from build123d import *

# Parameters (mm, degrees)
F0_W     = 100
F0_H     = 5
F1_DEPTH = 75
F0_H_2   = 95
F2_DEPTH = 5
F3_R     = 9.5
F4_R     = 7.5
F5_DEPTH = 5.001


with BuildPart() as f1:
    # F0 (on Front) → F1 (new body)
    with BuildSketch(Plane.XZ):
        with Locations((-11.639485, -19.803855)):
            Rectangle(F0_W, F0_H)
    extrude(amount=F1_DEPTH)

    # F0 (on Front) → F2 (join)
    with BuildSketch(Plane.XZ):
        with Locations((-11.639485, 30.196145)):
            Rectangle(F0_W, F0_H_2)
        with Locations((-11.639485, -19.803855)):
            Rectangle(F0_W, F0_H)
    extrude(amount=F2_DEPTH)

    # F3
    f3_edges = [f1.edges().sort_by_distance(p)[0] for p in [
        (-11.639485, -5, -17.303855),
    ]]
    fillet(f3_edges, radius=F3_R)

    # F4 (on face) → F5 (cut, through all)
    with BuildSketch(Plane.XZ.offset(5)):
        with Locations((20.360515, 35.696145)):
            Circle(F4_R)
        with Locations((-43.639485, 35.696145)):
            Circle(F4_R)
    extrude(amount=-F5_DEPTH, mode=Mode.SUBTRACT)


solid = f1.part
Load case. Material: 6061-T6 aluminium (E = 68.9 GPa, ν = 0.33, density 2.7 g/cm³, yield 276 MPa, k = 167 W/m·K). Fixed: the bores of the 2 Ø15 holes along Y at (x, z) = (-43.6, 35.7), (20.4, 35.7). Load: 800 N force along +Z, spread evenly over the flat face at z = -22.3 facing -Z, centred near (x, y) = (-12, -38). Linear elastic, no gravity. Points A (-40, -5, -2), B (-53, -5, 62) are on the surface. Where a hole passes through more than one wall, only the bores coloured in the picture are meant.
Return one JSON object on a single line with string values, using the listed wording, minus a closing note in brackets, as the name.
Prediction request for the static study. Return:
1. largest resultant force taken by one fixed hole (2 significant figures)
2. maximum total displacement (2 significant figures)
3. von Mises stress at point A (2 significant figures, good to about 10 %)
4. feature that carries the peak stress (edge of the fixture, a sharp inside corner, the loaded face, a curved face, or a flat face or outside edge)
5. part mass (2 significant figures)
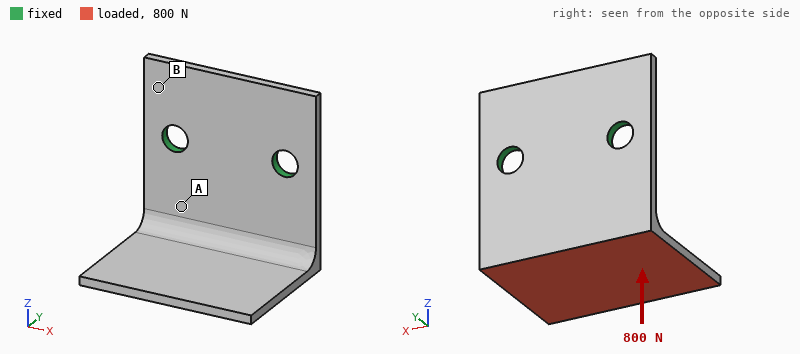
{"largest resultant force taken by one fixed hole": "410 N", "maximum total displacement": "1.6 mm", "von Mises stress at point A": "61 MPa", "feature that carries the peak stress": "a flat face or outside edge", "part mass": "230 g"}
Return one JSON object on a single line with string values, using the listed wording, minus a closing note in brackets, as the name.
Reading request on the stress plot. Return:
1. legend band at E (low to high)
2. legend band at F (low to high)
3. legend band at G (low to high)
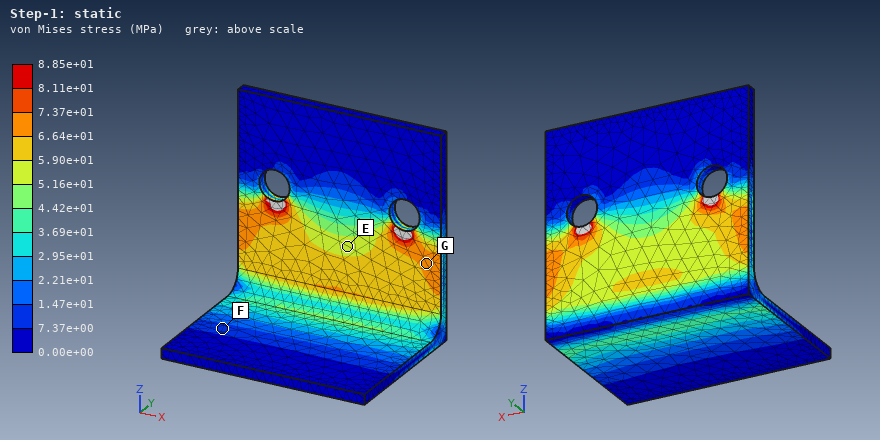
{"legend band at E": "5.16e+01 to 5.90e+01 MPa", "legend band at F": "7.37e+00 to 1.47e+01 MPa", "legend band at G": "6.64e+01 to 7.37e+01 MPa"}
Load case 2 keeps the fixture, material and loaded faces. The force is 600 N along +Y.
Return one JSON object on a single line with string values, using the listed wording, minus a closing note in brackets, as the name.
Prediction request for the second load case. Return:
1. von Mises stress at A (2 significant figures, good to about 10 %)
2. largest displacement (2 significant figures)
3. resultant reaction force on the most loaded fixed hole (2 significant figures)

{"von Mises stress at A": "26 MPa", "largest displacement": "0.93 mm", "resultant reaction force on the most loaded fixed hole": "300 N"}
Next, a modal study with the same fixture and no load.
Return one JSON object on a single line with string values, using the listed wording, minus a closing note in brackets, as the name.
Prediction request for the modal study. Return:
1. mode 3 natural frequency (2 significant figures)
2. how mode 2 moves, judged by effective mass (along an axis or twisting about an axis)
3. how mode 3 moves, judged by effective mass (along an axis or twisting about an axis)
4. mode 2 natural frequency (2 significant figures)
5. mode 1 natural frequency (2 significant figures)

{"mode 3 natural frequency": "1100 Hz", "how mode 2 moves, judged by effective mass": "along X", "how mode 3 moves, judged by effective mass": "along Y", "mode 2 natural frequency": "760 Hz", "mode 1 natural frequency": "380 Hz"}
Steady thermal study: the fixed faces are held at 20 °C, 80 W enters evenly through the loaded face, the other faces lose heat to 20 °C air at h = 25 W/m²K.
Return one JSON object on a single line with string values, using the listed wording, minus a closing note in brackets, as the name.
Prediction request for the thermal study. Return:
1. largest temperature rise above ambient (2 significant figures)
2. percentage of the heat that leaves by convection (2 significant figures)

{"largest temperature rise above ambient": "64 K", "percentage of the heat that leaves by convection": "22 %"}
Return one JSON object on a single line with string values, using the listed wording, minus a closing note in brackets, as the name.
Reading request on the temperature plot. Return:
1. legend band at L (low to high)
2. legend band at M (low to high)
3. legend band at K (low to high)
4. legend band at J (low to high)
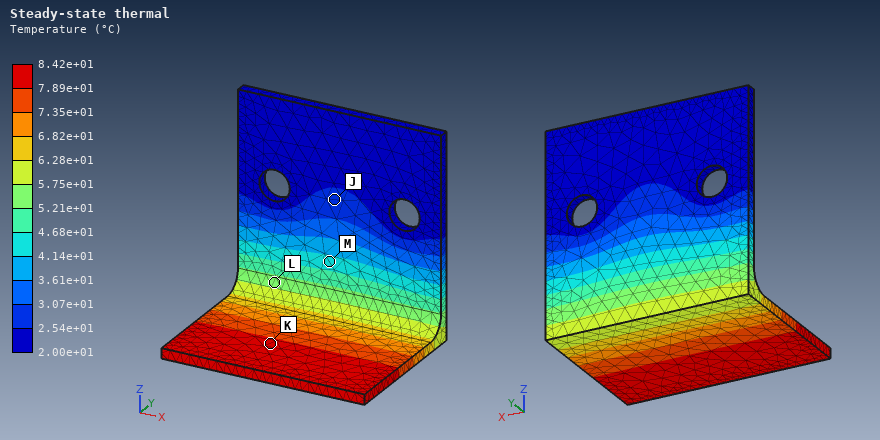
{"legend band at L": "5.21e+01 to 5.75e+01 °C", "legend band at M": "4.14e+01 to 4.68e+01 °C", "legend band at K": "7.89e+01 to 8.42e+01 °C", "legend band at J": "2.54e+01 to 3.07e+01 °C"}
